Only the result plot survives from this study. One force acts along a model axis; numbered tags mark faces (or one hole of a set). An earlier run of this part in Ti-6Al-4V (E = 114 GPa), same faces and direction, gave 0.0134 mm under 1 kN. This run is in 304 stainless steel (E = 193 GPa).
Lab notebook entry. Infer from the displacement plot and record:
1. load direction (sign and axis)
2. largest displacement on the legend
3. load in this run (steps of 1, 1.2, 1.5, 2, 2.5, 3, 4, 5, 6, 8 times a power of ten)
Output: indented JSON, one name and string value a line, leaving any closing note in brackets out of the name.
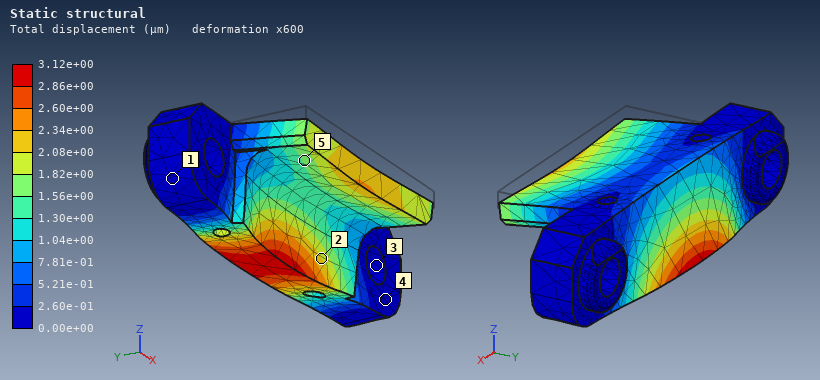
{
  "load direction": "+Y",
  "largest displacement on the legend": "3.12e+00 µm",
  "load in this run": "400 N"
}
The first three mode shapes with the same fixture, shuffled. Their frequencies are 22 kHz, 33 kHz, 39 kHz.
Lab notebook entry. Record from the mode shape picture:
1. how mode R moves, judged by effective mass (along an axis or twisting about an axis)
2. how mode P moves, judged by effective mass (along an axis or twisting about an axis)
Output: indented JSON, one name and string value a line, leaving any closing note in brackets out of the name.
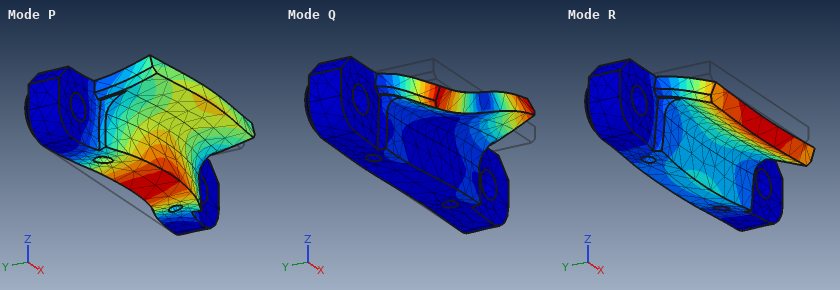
{
  "how mode R moves, judged by effective mass": "along Z",
  "how mode P moves, judged by effective mass": "along Y"
}
